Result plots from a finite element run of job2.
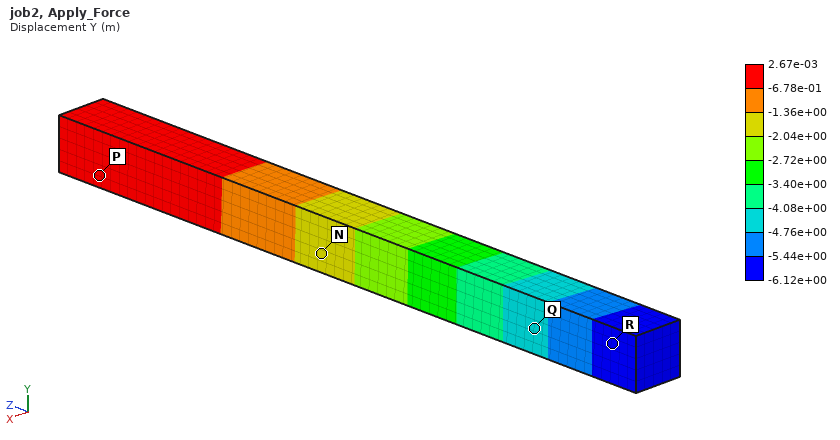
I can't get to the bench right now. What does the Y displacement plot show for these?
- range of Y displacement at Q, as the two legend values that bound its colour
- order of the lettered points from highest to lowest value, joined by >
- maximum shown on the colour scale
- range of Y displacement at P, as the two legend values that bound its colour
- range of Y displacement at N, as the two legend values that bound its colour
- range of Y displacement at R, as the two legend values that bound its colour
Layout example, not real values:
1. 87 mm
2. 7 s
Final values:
1. -4.76e+00 to -4.08e+00 m
2. P > N > Q > R
3. 2.67e-03 m
4. -6.78e-01 to 2.67e-03 m
5. -2.04e+00 to -1.36e+00 m
6. -6.12e+00 to -5.44e+00 m
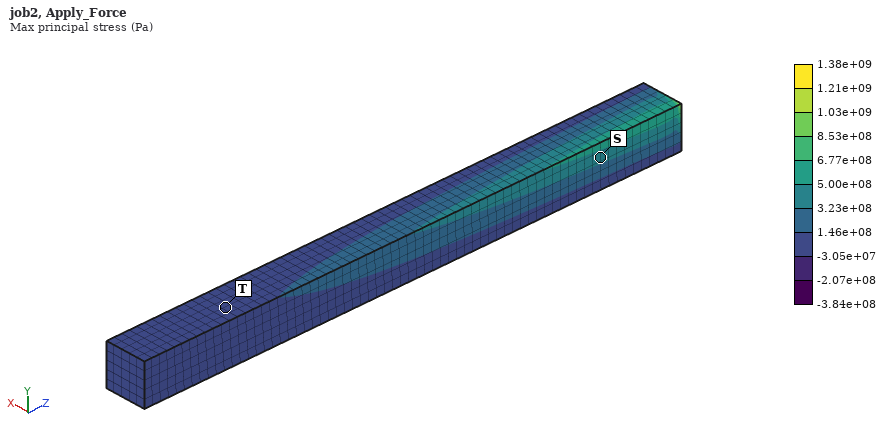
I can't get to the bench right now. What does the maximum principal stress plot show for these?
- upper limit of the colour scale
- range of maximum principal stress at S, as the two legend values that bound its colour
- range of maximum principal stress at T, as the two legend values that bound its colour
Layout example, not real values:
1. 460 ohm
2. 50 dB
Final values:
1. 1.38e+09 Pa
2. 3.23e+08 to 5.00e+08 Pa
3. -3.05e+07 to 1.46e+08 Pa
